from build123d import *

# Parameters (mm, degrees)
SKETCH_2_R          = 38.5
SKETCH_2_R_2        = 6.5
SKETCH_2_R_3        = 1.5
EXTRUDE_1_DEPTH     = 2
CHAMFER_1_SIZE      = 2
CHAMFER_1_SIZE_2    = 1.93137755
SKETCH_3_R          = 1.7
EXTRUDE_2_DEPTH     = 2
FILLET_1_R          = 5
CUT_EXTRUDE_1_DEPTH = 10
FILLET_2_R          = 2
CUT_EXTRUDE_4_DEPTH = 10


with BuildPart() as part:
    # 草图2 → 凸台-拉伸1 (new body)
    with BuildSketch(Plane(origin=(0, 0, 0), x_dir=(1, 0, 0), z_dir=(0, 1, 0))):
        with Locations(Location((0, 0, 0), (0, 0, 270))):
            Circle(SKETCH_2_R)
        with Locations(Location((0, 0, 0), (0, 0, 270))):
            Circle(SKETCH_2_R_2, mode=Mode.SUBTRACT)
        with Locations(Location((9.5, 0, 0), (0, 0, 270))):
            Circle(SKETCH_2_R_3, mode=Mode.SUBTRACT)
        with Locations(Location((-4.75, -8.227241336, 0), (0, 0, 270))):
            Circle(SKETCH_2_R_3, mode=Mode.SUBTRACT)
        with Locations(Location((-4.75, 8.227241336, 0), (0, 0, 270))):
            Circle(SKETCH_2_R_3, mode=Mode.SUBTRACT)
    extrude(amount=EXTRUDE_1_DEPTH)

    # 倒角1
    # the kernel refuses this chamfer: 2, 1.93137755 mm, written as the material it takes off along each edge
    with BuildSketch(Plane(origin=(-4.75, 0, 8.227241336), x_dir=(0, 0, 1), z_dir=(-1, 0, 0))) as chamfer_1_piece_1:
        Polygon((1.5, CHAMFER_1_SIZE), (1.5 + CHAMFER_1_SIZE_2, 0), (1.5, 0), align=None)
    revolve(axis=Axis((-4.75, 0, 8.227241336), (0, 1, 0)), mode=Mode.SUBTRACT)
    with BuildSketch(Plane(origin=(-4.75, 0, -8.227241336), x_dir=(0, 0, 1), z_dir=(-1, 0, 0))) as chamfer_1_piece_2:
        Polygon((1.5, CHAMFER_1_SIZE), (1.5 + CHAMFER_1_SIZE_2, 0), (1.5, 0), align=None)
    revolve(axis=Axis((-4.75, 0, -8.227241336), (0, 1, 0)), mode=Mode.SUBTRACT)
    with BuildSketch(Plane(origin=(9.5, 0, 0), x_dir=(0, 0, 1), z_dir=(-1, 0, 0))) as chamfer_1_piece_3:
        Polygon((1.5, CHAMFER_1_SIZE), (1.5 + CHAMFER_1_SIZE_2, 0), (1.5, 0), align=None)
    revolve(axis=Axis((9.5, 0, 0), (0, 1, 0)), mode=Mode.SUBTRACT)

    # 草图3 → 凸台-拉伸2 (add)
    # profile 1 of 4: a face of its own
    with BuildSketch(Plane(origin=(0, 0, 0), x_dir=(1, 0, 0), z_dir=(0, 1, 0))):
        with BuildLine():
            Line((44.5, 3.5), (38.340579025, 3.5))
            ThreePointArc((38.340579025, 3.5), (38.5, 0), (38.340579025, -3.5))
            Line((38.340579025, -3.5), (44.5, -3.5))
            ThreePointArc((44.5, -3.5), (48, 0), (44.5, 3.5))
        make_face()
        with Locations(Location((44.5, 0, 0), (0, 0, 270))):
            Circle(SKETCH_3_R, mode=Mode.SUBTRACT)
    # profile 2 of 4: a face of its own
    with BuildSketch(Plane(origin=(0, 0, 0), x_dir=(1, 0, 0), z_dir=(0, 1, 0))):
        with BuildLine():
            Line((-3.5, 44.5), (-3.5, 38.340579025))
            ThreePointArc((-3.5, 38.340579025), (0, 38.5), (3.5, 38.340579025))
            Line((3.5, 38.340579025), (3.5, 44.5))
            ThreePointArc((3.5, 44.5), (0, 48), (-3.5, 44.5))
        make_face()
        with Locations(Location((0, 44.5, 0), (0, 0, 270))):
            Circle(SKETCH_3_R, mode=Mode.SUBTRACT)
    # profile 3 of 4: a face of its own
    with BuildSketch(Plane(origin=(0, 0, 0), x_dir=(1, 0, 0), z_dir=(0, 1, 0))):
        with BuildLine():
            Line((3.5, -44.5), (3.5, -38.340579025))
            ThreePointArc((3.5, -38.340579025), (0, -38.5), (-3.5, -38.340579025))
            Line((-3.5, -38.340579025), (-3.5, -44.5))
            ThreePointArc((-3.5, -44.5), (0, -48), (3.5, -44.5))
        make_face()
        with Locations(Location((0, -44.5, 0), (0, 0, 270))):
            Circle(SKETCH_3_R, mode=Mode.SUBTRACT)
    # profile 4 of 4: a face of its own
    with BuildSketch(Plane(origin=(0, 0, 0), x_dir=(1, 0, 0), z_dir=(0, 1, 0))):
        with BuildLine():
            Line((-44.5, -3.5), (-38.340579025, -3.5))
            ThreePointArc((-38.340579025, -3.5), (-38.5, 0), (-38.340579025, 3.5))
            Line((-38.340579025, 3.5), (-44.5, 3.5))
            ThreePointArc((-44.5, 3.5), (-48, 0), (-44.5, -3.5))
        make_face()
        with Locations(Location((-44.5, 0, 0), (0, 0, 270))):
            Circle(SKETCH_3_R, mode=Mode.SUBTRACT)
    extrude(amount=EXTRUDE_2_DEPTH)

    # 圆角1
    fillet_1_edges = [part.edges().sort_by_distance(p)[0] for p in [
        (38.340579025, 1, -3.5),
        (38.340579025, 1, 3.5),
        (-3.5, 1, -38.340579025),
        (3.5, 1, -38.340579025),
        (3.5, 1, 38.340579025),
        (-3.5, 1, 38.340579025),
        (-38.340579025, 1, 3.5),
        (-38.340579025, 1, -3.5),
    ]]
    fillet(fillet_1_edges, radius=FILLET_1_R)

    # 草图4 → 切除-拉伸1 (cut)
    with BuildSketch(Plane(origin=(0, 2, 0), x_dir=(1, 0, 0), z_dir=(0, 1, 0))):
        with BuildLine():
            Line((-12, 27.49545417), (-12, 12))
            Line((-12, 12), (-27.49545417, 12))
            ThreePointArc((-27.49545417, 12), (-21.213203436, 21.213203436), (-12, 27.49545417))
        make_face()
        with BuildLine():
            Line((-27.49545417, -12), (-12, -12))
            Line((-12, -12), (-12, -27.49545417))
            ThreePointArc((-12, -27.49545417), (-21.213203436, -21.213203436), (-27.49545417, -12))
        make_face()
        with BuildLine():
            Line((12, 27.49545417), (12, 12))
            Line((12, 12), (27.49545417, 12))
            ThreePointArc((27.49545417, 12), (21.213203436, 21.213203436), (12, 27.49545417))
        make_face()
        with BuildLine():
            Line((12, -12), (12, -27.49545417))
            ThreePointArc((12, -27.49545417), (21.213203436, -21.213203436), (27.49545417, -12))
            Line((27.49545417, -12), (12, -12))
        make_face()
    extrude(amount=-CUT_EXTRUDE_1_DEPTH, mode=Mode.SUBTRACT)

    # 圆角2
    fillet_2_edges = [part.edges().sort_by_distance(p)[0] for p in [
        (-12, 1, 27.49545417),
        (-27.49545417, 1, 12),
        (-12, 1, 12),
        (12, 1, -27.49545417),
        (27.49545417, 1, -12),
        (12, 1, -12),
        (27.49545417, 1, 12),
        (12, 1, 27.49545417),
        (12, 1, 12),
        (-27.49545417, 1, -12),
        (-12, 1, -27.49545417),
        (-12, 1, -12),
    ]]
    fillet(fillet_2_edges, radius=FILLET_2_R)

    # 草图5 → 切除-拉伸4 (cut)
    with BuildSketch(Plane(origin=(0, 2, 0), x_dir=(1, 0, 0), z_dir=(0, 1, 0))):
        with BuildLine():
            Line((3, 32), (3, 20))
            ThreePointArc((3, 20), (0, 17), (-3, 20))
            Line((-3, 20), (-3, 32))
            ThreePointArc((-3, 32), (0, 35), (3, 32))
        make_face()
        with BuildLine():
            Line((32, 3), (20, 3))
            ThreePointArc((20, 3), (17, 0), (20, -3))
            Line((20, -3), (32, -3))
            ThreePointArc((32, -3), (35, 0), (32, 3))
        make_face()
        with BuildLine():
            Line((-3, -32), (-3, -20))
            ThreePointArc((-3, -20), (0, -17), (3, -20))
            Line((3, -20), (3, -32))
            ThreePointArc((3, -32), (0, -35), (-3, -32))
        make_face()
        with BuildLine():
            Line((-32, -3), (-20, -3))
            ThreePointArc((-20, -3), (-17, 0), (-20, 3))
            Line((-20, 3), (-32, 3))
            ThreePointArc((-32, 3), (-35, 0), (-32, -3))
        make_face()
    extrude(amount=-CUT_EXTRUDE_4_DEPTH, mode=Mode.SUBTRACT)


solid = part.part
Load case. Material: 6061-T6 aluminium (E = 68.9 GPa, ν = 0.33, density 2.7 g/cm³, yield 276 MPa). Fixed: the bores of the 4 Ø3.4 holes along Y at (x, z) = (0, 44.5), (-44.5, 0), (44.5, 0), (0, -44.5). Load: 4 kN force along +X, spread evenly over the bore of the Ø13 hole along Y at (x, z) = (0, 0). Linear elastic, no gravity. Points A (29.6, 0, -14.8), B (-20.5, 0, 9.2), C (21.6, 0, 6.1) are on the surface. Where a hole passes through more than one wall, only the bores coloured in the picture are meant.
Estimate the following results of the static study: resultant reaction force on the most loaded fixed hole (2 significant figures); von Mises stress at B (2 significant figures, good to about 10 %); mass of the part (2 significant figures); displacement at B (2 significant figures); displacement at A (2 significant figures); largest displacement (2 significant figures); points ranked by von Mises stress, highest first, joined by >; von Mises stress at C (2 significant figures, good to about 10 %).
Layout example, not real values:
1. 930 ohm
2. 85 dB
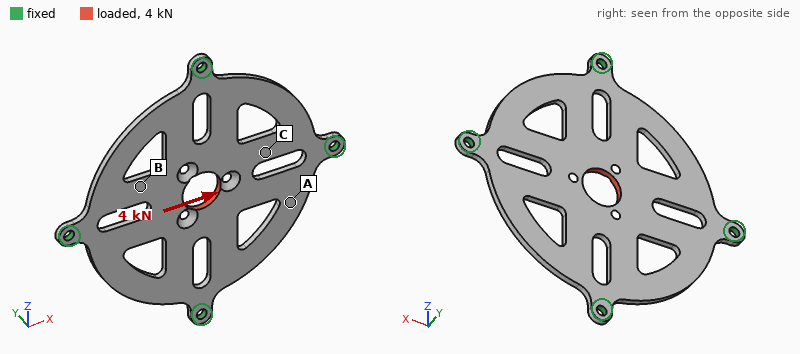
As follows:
1. 1.6 kN
2. 41 MPa
3. 20 g
4. 31 µm
5. 30 µm
6. 70 µm
7. C > B > A
8. 55 MPa
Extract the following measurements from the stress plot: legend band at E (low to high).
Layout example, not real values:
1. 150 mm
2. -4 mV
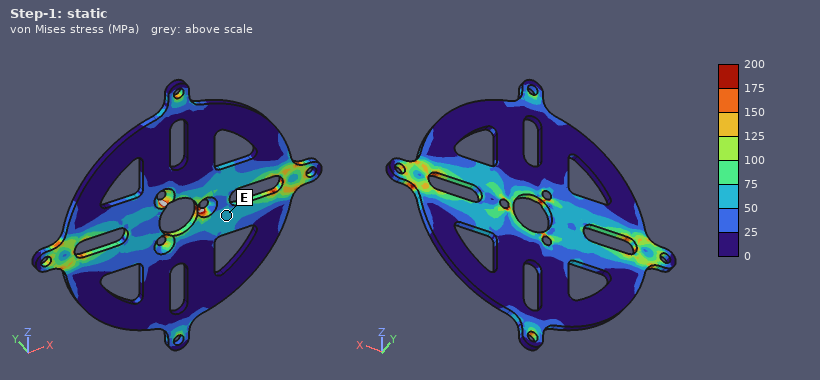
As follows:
1. 50 to 75 MPa
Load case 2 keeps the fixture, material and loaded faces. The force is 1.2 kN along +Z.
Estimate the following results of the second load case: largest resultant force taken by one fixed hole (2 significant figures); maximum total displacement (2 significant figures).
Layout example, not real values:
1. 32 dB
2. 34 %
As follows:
1. 470 N
2. 21 µm
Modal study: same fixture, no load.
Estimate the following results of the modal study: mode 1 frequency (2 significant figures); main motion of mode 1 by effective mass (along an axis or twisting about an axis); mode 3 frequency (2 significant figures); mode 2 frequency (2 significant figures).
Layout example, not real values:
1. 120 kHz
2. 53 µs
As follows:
1. 1500 Hz
2. along Y
3. 2500 Hz
4. 2500 Hz
